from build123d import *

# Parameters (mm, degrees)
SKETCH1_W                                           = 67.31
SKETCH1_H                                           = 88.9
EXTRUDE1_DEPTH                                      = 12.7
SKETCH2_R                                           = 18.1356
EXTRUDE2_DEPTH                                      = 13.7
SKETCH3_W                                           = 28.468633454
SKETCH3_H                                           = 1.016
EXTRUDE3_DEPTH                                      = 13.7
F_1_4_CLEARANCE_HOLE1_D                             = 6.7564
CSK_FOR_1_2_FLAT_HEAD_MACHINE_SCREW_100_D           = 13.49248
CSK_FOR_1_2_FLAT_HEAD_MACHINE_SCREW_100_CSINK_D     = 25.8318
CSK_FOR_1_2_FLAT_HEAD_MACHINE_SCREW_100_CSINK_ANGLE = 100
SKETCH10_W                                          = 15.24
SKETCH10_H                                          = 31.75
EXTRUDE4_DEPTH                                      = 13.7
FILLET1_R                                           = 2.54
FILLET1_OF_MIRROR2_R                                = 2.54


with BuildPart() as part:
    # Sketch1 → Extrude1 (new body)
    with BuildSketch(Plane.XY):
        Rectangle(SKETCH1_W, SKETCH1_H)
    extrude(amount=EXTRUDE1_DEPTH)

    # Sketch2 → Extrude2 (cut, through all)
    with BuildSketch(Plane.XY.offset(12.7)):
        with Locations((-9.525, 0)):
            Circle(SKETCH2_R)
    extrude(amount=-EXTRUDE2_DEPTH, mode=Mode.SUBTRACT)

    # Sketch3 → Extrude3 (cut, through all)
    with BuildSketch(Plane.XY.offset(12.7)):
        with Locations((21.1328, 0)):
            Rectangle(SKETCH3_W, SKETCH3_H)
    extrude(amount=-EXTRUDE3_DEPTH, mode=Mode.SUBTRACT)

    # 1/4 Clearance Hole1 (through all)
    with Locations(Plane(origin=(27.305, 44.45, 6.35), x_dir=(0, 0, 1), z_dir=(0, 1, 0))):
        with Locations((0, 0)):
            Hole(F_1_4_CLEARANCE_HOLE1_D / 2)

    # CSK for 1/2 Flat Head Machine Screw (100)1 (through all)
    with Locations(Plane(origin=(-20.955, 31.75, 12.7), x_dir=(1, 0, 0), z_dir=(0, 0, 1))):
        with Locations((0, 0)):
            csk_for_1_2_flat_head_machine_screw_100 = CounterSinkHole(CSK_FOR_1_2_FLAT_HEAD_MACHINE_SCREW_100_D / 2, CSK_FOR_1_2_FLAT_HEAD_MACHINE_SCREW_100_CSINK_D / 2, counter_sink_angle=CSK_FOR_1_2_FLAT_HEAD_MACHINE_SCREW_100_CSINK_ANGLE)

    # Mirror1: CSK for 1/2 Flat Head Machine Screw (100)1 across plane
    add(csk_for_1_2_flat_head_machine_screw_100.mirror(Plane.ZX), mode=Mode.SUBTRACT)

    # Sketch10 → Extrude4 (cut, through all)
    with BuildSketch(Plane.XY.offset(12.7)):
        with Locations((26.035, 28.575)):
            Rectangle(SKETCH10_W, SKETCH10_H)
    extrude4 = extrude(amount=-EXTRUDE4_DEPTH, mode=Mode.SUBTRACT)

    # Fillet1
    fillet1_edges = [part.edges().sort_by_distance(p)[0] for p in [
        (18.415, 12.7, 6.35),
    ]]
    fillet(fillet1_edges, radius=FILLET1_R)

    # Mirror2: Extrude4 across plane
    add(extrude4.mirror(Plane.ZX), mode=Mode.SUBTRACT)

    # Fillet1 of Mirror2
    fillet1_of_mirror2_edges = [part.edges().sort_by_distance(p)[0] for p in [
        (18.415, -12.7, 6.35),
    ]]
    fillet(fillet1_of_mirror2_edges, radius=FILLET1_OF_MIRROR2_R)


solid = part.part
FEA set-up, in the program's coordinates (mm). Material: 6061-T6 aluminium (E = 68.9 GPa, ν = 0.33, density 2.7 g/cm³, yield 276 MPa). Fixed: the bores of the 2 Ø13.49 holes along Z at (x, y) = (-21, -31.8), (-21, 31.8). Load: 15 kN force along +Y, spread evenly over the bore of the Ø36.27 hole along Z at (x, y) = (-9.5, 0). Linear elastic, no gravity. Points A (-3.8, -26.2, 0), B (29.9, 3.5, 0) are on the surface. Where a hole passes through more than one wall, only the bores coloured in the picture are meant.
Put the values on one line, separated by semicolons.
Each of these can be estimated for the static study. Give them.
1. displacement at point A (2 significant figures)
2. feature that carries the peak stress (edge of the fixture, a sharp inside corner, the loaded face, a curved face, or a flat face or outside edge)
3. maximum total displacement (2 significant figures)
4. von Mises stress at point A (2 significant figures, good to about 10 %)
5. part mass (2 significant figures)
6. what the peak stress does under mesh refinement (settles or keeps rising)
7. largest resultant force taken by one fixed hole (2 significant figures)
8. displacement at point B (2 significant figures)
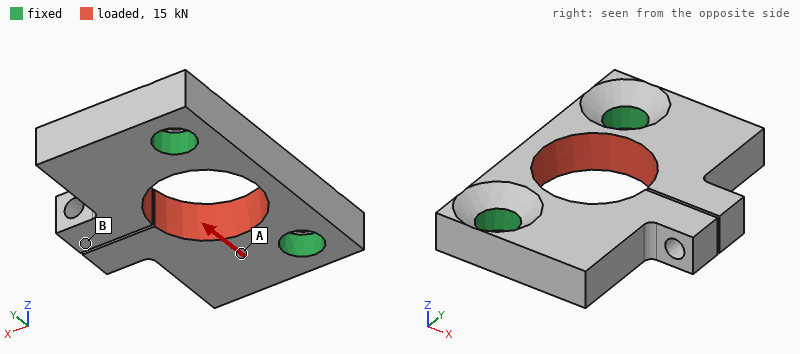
17 µm; edge of the fixture; 61 µm; 26 MPa; 120 g; keeps rising; 7.5 kN; 56 µm
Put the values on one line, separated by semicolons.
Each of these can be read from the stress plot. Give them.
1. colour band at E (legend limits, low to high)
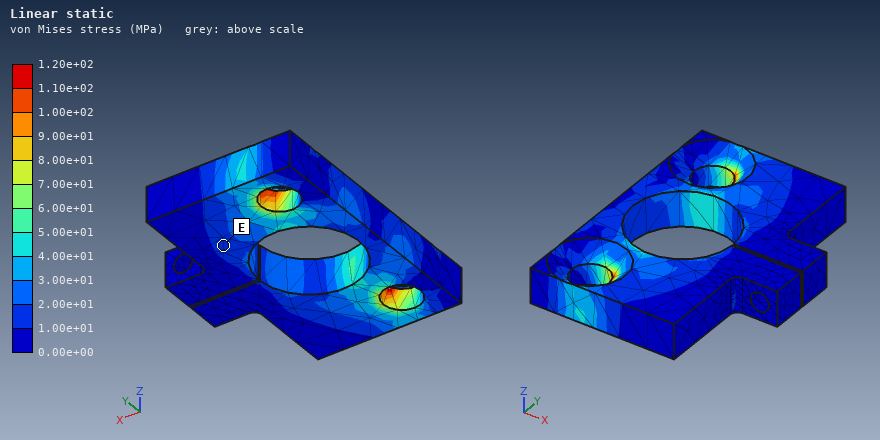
1.00e+01 to 2.00e+01 MPa
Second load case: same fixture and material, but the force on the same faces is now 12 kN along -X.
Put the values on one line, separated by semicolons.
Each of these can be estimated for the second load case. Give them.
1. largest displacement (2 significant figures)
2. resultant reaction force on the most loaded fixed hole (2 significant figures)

0.11 mm; 6.3 kN
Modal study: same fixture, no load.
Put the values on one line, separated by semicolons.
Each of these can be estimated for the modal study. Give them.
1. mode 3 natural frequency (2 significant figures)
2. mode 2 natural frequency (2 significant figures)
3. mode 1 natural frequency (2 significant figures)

5700 Hz; 3300 Hz; 3300 Hz
